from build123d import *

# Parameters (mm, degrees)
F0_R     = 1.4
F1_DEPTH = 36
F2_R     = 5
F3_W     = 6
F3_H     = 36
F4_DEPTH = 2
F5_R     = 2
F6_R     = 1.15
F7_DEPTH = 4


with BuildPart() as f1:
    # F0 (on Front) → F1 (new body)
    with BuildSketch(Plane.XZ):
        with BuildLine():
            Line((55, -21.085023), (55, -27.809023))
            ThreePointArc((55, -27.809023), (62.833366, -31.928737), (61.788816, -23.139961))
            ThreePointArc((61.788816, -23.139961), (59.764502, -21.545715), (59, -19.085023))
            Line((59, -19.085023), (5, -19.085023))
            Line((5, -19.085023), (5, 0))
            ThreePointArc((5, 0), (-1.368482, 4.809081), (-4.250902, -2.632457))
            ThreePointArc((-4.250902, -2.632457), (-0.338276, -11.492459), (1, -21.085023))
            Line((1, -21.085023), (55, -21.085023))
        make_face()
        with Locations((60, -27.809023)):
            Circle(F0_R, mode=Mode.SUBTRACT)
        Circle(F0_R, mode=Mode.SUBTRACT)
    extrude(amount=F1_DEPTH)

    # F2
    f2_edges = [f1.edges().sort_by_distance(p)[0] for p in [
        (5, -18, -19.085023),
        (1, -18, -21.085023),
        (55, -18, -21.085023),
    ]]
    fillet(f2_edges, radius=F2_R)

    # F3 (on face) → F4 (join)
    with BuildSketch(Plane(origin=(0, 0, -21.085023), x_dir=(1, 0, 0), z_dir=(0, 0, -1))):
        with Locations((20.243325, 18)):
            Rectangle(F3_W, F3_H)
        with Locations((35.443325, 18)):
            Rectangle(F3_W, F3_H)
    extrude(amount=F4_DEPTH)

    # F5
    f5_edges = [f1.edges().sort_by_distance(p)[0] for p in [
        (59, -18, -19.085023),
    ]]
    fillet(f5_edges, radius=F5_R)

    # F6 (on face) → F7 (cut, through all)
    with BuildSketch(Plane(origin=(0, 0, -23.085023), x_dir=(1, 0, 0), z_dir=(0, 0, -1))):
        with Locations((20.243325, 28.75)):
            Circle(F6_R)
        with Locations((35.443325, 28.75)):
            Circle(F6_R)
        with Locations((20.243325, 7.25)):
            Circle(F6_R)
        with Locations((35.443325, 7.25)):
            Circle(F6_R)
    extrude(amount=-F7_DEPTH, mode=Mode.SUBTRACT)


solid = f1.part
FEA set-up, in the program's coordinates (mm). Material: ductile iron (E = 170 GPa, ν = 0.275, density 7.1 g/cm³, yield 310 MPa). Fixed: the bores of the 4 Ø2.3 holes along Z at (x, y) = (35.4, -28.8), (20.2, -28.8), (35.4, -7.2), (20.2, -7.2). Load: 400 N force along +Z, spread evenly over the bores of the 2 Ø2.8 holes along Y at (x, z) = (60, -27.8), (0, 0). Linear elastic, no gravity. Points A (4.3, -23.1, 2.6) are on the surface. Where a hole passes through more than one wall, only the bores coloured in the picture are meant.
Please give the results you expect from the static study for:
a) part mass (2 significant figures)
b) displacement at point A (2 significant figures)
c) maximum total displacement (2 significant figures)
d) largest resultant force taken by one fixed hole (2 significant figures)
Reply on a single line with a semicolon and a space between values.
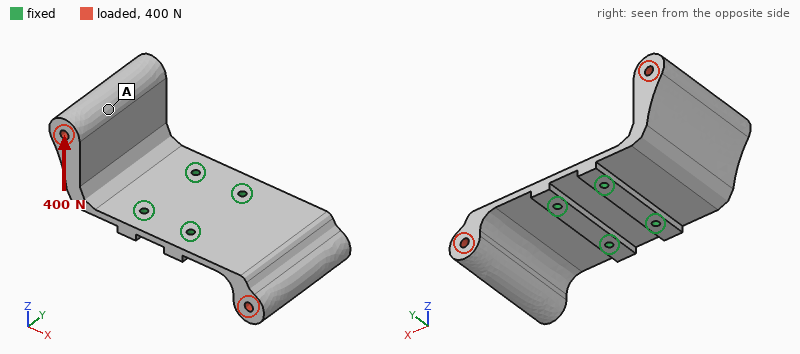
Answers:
99 g; 0.17 mm; 0.26 mm; 170 N
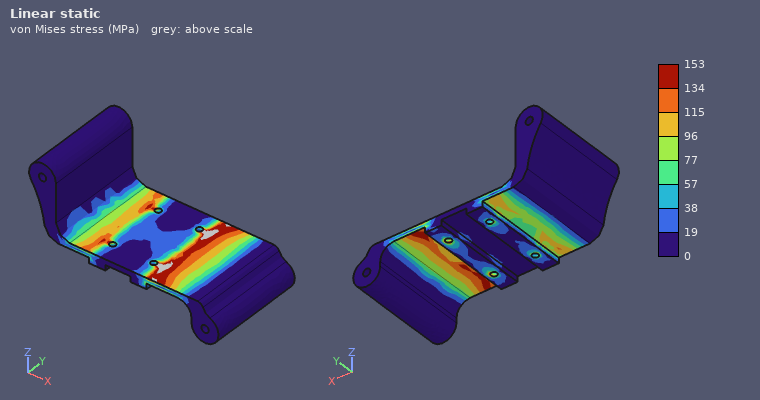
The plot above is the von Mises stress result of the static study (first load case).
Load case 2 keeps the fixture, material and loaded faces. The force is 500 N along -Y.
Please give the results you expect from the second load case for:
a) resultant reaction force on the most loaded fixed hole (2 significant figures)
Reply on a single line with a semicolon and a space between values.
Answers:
290 N
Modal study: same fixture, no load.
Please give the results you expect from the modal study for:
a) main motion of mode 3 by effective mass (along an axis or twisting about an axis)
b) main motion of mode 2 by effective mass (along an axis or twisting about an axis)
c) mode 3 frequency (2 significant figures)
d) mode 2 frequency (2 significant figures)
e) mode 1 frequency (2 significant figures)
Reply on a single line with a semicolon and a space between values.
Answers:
along Y; along Z; 2200 Hz; 980 Hz; 770 Hz
